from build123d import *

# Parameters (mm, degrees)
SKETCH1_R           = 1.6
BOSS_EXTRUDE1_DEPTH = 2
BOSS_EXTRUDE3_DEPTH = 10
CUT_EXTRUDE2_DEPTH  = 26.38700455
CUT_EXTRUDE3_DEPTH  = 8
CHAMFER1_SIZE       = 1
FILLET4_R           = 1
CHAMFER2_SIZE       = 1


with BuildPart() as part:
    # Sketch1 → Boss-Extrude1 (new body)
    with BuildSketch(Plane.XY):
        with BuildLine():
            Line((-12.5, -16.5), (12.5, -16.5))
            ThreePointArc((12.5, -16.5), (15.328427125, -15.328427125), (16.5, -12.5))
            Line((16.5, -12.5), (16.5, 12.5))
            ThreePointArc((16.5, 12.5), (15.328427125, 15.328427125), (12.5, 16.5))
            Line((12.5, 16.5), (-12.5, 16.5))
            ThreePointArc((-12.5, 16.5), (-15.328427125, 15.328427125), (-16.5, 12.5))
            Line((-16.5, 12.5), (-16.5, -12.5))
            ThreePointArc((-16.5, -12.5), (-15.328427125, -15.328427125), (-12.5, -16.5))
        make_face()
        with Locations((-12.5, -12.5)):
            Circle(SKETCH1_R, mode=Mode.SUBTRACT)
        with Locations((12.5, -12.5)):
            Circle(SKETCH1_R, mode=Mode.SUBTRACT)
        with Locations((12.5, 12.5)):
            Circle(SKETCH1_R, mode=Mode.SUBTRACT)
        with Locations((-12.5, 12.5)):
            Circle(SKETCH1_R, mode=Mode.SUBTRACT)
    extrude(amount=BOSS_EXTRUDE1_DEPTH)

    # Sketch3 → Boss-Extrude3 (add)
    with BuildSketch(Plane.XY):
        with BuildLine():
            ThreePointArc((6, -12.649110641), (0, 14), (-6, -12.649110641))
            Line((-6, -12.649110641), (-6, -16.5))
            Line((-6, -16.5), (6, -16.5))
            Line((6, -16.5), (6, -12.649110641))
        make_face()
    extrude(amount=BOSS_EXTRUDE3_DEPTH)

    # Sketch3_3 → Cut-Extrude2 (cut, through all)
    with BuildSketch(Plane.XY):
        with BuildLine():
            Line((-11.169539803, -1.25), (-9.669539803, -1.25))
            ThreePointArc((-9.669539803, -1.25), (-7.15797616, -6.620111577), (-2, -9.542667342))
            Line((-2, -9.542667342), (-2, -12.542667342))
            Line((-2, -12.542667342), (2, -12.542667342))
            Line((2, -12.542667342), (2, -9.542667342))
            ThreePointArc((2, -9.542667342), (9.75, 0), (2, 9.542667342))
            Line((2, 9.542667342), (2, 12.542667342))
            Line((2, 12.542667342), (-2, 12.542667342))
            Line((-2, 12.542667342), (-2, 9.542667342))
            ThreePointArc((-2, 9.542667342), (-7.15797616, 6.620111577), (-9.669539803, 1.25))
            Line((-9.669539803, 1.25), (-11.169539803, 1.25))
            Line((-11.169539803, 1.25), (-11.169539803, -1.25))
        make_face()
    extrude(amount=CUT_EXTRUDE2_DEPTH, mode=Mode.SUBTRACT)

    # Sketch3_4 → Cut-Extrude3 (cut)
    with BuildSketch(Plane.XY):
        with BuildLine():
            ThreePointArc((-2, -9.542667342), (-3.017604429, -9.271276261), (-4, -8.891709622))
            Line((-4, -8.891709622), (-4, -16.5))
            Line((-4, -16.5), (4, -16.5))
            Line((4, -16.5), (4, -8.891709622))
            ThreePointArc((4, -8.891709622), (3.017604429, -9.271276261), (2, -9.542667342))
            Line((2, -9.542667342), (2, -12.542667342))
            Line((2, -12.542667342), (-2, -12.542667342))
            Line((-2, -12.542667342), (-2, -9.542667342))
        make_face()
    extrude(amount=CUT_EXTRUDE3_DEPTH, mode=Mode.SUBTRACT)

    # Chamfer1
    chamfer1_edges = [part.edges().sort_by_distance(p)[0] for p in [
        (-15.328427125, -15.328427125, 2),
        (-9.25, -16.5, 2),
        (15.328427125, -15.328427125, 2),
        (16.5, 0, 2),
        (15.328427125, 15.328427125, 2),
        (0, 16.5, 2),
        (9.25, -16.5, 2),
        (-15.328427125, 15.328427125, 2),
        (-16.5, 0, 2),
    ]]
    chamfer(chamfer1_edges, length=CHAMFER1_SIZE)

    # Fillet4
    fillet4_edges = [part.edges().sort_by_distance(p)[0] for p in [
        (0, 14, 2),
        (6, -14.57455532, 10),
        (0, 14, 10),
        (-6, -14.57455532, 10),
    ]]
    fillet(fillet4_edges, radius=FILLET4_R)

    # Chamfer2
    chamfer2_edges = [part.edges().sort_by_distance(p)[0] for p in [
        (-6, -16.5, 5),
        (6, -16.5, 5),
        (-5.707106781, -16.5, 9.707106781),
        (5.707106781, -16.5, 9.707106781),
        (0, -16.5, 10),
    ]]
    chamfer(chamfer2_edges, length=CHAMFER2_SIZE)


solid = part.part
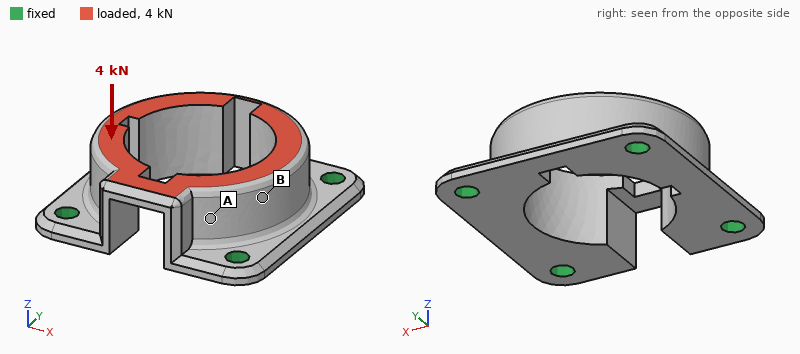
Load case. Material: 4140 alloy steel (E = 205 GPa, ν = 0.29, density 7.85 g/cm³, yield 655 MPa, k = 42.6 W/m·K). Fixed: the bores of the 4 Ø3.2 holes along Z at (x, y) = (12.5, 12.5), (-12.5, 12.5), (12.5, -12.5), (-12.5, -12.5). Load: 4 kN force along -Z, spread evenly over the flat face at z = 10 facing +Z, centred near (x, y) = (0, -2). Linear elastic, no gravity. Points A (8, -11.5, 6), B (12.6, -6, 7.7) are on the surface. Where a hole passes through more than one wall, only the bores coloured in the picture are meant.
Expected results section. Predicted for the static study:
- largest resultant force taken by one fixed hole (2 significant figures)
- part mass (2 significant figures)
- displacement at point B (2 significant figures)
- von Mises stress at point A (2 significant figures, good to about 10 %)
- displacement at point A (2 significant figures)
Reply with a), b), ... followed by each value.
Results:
a) 1.3 kN
b) 28 g
c) 8.2 µm
d) 66 MPa
e) 9.9 µm
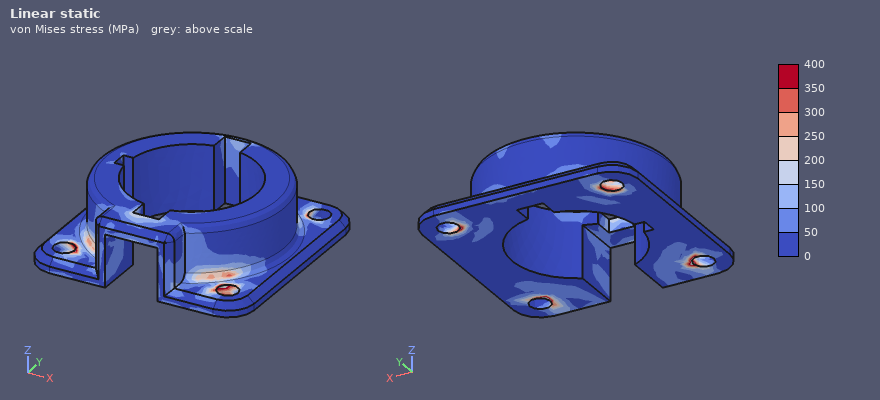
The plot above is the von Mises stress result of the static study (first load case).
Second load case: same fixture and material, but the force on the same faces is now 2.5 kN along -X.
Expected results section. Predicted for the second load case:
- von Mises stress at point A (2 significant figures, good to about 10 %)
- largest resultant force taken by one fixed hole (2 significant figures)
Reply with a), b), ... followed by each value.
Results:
a) 51 MPa
b) 940 N
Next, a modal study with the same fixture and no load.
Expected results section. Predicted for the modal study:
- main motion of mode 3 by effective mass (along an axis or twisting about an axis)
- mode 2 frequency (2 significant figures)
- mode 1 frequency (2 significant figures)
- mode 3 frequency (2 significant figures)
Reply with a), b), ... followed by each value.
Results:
a) along Z
b) 18 kHz
c) 18 kHz
d) 22 kHz
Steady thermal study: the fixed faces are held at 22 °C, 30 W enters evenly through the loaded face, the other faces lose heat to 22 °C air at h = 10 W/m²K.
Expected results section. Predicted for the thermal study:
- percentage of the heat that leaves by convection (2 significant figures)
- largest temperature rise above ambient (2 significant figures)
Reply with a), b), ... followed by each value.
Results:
a) 3.2 %
b) 76 K
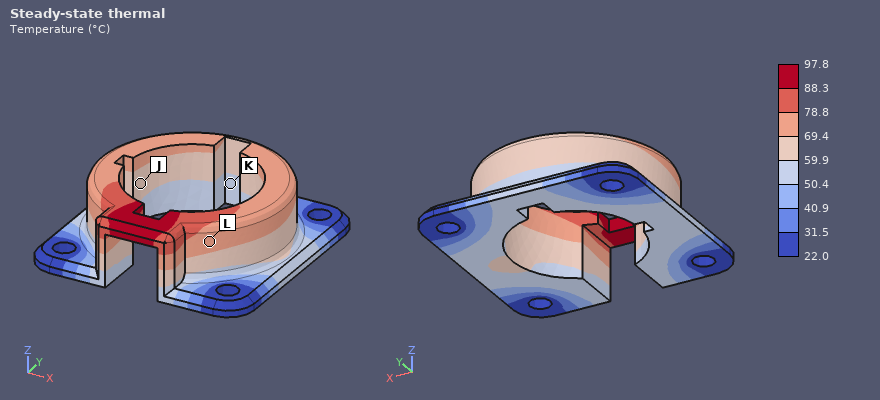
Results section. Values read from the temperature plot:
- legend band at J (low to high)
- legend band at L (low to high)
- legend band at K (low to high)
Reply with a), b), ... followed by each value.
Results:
a) 59.9 to 69.4 °C
b) 69.4 to 78.8 °C
c) 50.4 to 59.9 °C
